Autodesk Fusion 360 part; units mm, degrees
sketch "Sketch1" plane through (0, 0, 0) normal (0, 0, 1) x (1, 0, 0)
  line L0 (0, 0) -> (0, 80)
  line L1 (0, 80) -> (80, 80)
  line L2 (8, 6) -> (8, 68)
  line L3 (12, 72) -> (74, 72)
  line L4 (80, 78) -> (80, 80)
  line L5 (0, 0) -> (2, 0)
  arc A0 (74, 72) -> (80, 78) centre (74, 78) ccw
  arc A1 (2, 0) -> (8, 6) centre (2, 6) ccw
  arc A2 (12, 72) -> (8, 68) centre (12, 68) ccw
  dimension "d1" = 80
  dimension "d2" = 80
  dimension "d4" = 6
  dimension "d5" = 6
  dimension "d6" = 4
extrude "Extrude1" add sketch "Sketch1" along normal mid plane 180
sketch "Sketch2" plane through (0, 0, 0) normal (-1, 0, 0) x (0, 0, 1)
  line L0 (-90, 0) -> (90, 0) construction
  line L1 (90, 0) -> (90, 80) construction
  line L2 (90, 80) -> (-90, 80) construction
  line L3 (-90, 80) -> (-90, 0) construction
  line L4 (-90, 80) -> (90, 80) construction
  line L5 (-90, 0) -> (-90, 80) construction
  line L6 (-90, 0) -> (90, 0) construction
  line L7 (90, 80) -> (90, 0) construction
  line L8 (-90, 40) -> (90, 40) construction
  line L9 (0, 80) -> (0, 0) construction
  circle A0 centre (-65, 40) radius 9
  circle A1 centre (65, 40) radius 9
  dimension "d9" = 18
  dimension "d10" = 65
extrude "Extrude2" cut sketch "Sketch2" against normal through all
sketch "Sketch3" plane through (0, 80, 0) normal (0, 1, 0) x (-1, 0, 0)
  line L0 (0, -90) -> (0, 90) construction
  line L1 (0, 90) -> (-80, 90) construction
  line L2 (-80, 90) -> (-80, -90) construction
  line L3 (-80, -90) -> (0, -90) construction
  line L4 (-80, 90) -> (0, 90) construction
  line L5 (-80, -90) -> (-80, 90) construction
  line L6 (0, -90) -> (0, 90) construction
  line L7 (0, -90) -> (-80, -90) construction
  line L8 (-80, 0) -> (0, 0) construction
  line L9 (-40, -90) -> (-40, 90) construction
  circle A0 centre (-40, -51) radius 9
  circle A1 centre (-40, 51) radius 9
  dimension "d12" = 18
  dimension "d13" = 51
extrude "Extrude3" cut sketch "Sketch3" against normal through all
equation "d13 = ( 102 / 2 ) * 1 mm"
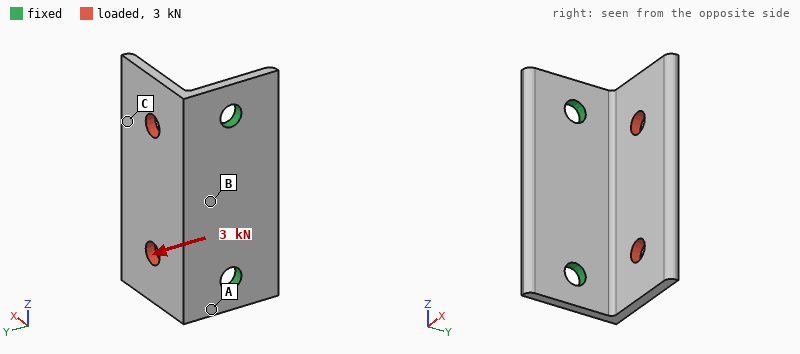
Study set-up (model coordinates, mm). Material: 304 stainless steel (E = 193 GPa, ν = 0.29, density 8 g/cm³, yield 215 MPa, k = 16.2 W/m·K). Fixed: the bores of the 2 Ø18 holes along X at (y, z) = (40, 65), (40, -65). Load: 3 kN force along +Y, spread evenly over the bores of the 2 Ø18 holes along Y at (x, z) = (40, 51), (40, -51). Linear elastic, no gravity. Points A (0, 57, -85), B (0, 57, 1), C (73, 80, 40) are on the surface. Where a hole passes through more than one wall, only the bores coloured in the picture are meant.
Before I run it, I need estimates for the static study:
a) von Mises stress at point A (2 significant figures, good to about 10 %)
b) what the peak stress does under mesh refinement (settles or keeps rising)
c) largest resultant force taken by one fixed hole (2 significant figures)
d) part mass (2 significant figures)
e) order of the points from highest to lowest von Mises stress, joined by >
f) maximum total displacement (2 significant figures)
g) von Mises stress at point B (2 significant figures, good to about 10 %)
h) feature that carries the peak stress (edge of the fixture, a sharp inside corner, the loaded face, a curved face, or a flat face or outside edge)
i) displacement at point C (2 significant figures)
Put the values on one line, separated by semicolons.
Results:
59 MPa; keeps rising; 1.5 kN; 1.7 kg; A > B > C; 0.25 mm; 33 MPa; edge of the fixture; 0.22 mm
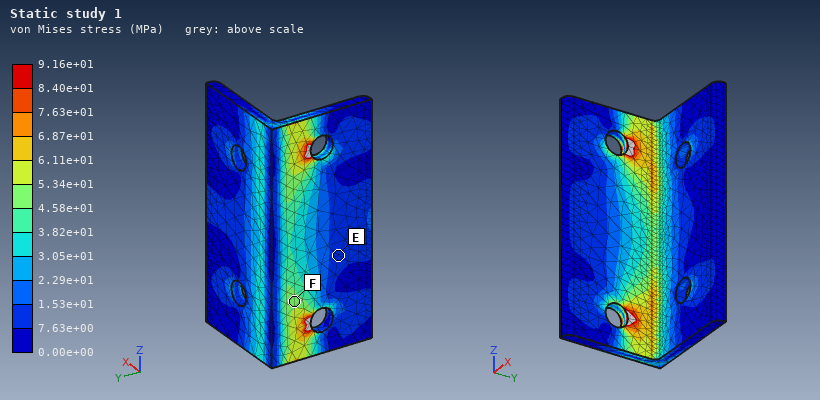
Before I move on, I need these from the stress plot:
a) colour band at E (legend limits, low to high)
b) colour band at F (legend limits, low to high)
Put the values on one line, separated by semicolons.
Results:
7.63e+00 to 1.53e+01 MPa; 4.58e+01 to 5.34e+01 MPa
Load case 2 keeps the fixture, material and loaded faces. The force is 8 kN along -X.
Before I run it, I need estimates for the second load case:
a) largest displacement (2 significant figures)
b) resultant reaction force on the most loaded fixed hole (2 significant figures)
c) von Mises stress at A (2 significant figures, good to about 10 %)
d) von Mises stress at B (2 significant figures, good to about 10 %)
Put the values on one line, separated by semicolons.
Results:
0.26 mm; 4.0 kN; 93 MPa; 30 MPa
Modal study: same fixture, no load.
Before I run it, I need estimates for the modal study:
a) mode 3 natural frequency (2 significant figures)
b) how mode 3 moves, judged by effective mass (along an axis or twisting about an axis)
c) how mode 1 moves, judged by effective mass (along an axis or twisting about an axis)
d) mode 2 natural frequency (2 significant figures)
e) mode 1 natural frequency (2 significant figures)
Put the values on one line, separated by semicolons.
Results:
2200 Hz; along X; along Y; 1200 Hz; 680 Hz
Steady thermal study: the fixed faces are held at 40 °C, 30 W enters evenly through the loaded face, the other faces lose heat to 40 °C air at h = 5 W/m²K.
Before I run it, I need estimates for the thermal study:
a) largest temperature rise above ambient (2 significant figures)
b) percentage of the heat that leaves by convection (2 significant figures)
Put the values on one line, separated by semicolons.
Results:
87 K; 36 %
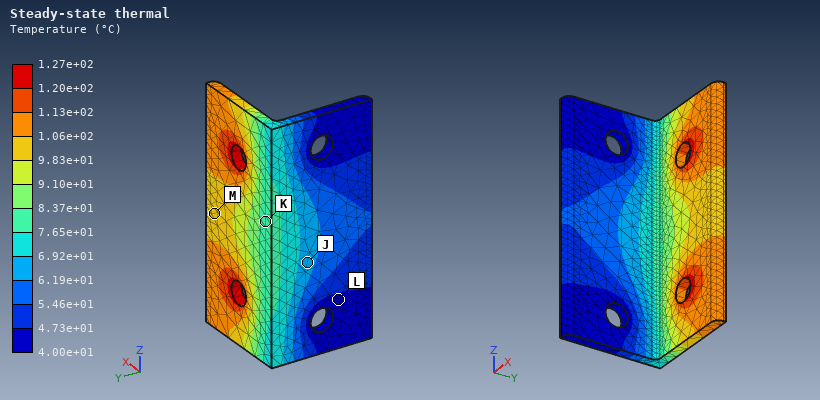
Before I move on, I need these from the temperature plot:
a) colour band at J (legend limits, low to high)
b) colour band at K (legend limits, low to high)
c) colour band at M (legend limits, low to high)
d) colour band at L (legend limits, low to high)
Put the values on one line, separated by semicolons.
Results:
6.19e+01 to 6.92e+01 °C; 7.65e+01 to 8.37e+01 °C; 9.83e+01 to 1.06e+02 °C; 4.00e+01 to 4.73e+01 °C
